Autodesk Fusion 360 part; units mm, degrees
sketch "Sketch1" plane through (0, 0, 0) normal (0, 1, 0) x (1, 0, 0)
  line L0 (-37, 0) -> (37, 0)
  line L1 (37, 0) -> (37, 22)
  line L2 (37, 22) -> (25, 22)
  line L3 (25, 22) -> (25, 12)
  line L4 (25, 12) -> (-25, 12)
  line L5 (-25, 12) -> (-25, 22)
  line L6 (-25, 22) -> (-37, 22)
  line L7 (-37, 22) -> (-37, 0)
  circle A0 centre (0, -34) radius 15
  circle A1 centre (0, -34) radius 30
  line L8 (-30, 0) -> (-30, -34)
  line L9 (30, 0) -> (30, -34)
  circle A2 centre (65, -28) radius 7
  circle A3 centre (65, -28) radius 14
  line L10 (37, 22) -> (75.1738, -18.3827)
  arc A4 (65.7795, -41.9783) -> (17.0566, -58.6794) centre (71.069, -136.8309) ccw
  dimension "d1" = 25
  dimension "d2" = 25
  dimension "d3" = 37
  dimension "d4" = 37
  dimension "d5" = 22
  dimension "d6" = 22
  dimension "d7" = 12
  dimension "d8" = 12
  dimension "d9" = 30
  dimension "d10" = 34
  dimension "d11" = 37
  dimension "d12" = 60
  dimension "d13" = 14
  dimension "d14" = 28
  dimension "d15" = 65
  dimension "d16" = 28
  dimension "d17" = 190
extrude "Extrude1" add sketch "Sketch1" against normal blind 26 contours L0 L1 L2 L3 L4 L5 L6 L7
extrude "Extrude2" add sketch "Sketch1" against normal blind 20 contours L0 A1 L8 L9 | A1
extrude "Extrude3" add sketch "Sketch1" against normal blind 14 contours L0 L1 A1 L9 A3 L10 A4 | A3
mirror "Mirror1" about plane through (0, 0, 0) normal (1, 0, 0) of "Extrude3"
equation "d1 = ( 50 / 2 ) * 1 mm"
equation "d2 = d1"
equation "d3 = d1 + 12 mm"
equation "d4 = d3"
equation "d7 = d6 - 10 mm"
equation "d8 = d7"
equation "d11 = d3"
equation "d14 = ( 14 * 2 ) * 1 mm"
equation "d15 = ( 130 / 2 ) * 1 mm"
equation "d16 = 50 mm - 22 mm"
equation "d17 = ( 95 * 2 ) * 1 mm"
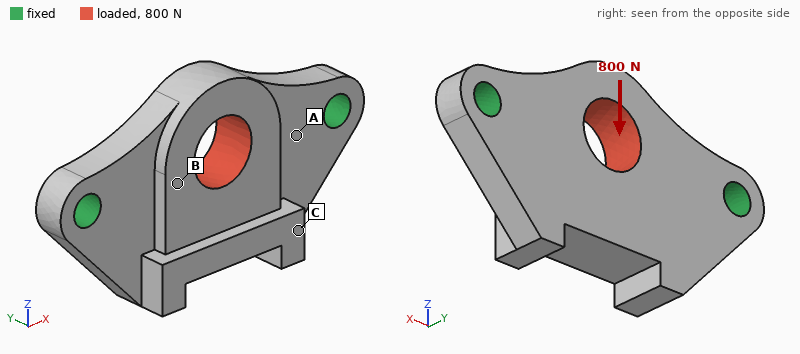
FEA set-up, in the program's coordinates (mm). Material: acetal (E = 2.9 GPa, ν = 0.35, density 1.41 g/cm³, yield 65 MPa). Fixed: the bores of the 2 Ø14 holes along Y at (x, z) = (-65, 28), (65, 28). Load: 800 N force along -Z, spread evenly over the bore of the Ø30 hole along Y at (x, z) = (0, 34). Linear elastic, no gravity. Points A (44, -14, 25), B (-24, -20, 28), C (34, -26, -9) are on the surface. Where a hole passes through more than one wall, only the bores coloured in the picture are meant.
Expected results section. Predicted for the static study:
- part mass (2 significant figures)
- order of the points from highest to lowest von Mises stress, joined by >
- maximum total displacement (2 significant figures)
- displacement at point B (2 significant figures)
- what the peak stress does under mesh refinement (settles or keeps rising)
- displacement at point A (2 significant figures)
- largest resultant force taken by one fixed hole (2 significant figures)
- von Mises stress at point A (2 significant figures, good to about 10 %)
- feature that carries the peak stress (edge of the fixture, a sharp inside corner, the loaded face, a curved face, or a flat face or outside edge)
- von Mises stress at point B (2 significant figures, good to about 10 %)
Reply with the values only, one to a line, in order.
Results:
200 g
A > B > C
78 µm
50 µm
keeps rising
23 µm
420 N
1.8 MPa
edge of the fixture
0.81 MPa
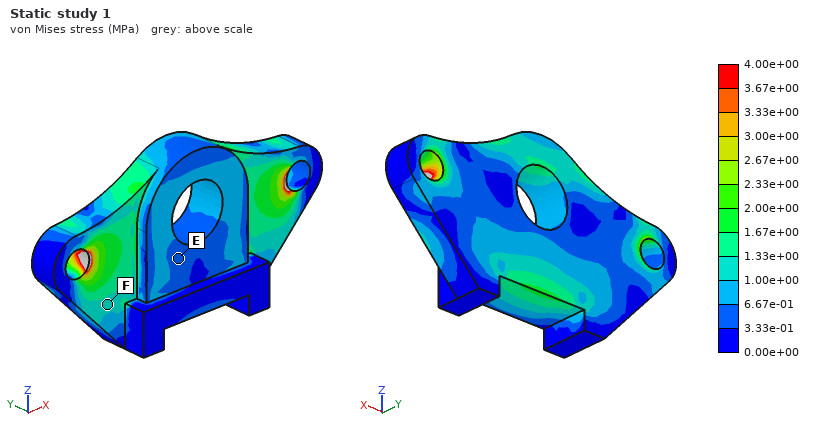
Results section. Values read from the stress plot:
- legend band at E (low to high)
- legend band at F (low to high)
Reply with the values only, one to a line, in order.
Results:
3.33e-01 to 6.67e-01 MPa
1.00e+00 to 1.33e+00 MPa
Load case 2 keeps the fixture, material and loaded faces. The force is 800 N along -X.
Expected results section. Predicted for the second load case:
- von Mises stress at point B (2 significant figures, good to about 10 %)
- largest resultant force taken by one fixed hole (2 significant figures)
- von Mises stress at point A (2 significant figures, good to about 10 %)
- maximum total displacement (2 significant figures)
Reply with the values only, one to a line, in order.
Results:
0.36 MPa
400 N
0.90 MPa
19 µm
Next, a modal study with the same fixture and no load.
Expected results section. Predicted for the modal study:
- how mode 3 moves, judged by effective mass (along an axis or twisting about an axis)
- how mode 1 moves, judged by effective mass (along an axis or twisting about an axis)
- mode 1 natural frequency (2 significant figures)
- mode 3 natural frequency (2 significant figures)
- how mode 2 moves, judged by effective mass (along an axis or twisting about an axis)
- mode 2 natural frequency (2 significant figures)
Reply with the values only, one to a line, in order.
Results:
twisting about Z
along Y
800 Hz
2000 Hz
along Y
1100 Hz
